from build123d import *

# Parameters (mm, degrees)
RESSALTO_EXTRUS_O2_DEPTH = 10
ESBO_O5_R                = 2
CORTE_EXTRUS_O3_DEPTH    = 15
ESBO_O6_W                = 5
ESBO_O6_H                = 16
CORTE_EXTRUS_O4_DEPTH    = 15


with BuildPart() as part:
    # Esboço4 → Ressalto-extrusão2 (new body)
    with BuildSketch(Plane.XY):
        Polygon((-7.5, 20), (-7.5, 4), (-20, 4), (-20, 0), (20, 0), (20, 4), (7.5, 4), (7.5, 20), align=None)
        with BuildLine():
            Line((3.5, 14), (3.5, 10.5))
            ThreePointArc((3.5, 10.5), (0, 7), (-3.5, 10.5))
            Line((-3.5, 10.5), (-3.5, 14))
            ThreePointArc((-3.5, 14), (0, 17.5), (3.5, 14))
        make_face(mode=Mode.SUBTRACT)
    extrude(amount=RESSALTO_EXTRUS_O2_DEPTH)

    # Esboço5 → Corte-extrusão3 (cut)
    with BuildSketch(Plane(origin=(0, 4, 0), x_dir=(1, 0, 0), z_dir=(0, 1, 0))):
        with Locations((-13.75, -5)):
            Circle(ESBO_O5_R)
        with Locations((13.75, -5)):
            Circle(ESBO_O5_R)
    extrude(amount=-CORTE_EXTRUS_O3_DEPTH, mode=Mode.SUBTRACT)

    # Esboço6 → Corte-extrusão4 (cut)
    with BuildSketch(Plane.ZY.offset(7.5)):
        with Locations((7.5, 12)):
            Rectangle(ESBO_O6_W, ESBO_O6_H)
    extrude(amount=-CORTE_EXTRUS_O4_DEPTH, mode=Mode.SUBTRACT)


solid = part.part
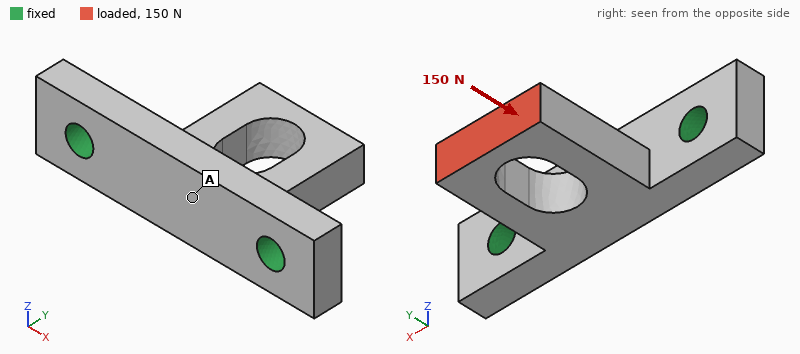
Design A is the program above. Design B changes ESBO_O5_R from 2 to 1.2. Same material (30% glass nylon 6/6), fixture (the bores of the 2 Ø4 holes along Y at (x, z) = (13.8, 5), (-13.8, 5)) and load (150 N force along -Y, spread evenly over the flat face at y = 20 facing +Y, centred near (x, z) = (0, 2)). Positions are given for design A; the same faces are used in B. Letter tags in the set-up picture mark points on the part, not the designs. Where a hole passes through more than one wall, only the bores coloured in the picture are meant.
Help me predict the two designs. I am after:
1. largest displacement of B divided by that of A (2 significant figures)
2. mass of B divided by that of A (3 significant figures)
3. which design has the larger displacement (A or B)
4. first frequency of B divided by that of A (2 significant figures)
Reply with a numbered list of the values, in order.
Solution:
1. 1.3
2. 1.03
3. B
4. 0.93
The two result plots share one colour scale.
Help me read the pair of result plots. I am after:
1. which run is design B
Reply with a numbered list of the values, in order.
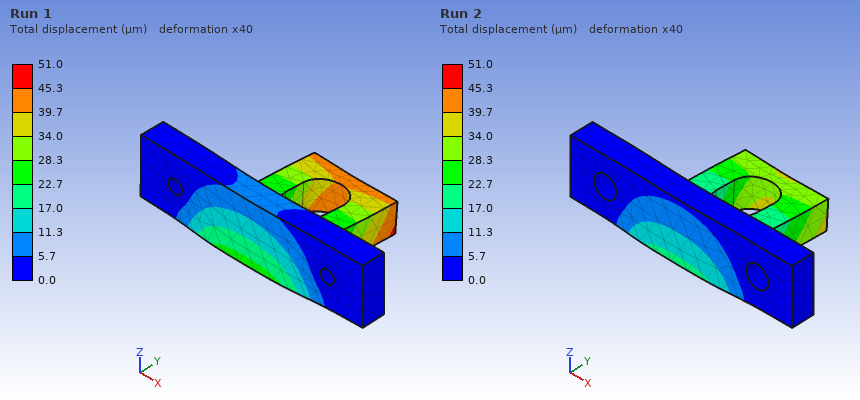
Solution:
1. Run 1
